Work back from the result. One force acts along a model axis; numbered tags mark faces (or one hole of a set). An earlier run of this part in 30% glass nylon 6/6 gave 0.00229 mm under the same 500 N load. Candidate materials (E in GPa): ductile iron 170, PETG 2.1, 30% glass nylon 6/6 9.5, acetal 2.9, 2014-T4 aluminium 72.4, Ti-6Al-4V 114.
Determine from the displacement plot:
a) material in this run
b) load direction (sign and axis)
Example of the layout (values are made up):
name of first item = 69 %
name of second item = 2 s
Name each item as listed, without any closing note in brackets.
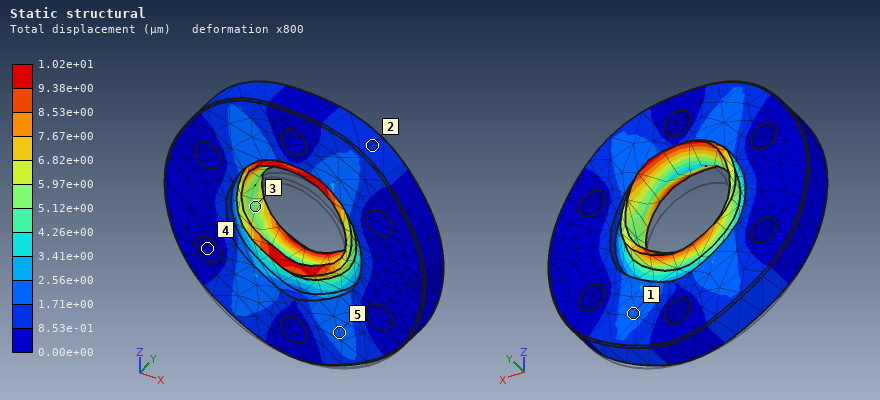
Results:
material in this run = PETG
load direction = +Z
